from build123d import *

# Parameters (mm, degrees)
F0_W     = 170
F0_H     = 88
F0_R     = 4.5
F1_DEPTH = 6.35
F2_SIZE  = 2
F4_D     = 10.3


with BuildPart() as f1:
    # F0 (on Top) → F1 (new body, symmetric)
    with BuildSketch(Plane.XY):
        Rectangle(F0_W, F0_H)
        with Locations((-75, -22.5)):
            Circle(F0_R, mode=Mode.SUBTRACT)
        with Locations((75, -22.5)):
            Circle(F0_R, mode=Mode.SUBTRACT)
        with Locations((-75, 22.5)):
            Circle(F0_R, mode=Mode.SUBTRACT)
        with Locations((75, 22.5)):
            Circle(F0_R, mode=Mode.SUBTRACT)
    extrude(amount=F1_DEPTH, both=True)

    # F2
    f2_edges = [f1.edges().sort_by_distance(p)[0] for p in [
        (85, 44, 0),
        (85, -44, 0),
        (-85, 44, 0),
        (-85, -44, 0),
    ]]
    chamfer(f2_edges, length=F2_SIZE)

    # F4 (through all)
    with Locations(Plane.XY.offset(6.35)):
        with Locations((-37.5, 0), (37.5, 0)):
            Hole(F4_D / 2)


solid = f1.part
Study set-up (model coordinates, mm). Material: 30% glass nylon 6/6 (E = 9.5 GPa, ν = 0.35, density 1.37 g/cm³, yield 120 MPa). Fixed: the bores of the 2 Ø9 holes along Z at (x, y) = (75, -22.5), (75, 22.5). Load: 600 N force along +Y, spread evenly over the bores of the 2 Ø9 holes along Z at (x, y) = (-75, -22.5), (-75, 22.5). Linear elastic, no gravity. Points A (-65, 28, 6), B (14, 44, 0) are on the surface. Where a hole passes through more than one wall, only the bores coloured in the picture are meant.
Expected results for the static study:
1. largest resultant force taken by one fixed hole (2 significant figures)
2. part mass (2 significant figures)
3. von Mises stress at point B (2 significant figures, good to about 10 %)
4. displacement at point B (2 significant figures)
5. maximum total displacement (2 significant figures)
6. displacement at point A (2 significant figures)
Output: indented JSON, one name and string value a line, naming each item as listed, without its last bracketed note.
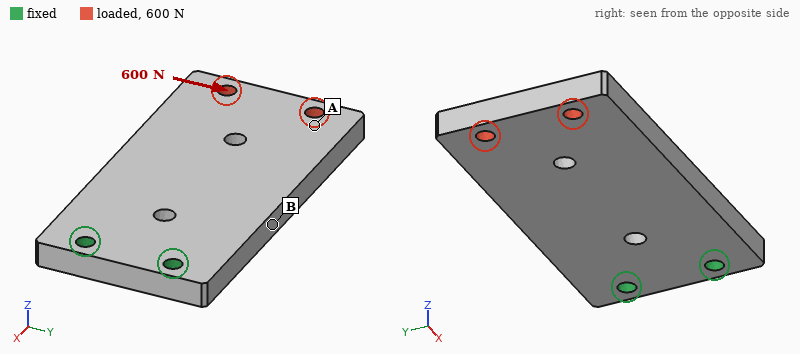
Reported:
{
  "largest resultant force taken by one fixed hole": "1.8 kN",
  "part mass": "250 g",
  "von Mises stress at point B": "3.1 MPa",
  "displacement at point B": "0.067 mm",
  "maximum total displacement": "0.19 mm",
  "displacement at point A": "0.16 mm"
}
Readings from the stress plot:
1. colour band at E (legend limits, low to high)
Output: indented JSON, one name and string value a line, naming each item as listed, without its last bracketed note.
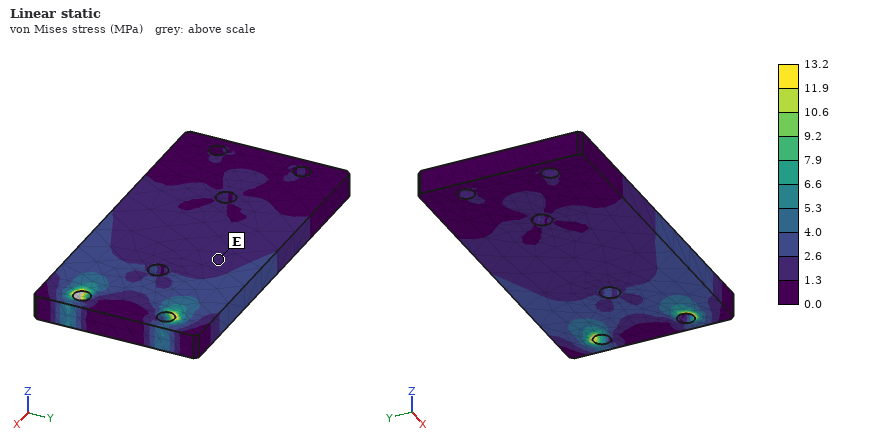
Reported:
{
  "colour band at E": "1.3 to 2.6 MPa"
}
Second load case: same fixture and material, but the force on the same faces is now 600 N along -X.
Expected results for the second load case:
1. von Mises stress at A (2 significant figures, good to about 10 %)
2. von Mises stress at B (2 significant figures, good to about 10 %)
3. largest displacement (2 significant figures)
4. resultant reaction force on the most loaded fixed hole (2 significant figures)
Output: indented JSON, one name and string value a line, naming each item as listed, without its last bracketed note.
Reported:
{
  "von Mises stress at A": "0.91 MPa",
  "von Mises stress at B": "0.56 MPa",
  "largest displacement": "12 µm",
  "resultant reaction force on the most loaded fixed hole": "300 N"
}
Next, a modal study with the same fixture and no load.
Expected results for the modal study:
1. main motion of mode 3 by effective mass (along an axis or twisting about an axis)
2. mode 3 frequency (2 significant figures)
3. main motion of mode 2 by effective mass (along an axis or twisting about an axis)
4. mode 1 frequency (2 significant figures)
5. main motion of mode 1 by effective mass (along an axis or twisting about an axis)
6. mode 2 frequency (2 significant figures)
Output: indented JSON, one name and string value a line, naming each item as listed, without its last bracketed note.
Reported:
{
  "main motion of mode 3 by effective mass": "along Y",
  "mode 3 frequency": "1000 Hz",
  "main motion of mode 2 by effective mass": "twisting about X",
  "mode 1 frequency": "210 Hz",
  "main motion of mode 1 by effective mass": "along Z",
  "mode 2 frequency": "770 Hz"
}
